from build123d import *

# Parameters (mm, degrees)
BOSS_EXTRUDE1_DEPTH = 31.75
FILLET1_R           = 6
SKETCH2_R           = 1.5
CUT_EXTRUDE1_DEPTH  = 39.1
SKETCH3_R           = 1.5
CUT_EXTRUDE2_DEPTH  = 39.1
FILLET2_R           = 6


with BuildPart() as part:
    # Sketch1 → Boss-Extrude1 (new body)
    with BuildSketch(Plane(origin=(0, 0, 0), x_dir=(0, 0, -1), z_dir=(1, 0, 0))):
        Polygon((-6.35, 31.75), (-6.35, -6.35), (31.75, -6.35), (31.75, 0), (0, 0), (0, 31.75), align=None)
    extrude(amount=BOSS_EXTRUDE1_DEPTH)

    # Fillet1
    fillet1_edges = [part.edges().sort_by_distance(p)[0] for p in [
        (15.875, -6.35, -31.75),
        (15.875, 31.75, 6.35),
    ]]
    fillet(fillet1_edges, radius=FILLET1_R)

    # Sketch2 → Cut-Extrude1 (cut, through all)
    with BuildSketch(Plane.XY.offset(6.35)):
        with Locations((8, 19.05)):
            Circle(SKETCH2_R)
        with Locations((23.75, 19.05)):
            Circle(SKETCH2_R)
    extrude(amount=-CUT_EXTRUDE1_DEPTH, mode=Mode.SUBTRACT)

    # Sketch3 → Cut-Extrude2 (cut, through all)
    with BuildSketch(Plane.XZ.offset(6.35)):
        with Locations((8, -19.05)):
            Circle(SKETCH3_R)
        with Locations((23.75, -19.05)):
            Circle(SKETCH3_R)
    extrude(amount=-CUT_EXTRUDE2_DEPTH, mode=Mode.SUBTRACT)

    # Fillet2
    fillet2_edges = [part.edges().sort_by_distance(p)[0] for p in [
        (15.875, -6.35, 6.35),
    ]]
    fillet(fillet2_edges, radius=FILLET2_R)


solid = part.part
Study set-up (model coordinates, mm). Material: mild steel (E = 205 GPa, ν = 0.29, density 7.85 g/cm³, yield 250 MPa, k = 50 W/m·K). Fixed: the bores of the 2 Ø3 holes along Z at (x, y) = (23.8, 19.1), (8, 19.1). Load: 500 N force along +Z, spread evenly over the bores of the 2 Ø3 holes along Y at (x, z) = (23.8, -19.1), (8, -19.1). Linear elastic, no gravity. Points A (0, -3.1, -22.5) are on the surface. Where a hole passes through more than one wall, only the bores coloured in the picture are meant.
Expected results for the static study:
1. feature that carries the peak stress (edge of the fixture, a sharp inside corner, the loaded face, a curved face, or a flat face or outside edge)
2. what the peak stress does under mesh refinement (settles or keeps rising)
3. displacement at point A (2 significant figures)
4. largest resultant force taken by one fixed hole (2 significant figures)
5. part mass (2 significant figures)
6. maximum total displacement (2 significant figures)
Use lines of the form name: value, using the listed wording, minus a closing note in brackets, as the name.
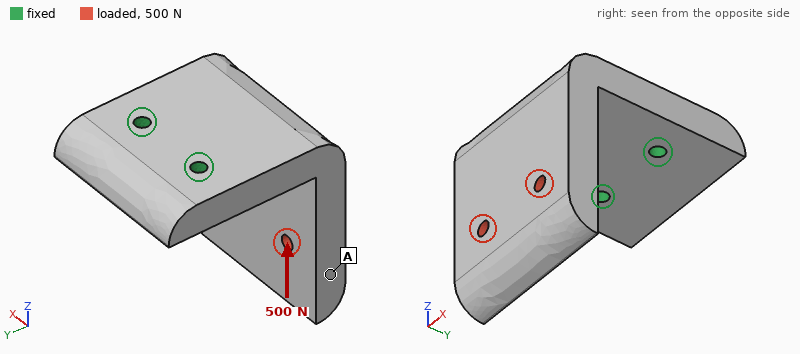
feature that carries the peak stress: edge of the fixture
what the peak stress does under mesh refinement: keeps rising
displacement at point A: 29 µm
largest resultant force taken by one fixed hole: 250 N
part mass: 100 g
maximum total displacement: 37 µm
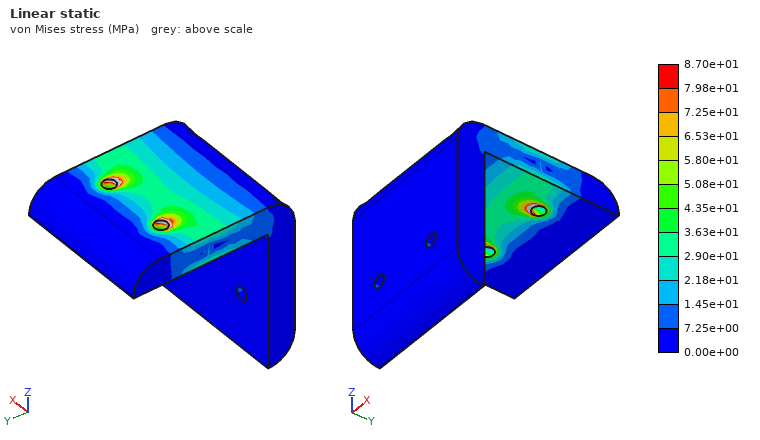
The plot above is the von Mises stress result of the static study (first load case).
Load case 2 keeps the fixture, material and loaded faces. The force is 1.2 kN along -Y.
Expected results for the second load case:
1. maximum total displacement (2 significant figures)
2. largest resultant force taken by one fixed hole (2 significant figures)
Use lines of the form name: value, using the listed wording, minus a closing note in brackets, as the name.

maximum total displacement: 0.20 mm
largest resultant force taken by one fixed hole: 610 N
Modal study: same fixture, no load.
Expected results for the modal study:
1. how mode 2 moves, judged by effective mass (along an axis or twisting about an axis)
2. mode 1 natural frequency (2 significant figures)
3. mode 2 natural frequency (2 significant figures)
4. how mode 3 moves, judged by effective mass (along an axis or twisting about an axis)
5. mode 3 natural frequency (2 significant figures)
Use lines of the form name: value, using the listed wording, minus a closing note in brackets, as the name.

how mode 2 moves, judged by effective mass: along X
mode 1 natural frequency: 2200 Hz
mode 2 natural frequency: 3600 Hz
how mode 3 moves, judged by effective mass: along Z
mode 3 natural frequency: 6200 Hz
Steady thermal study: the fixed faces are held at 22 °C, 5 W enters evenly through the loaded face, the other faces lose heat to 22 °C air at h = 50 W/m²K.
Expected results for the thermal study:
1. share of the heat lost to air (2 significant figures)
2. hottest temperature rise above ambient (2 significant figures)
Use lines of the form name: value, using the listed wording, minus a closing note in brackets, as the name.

share of the heat lost to air: 39 %
hottest temperature rise above ambient: 16 K
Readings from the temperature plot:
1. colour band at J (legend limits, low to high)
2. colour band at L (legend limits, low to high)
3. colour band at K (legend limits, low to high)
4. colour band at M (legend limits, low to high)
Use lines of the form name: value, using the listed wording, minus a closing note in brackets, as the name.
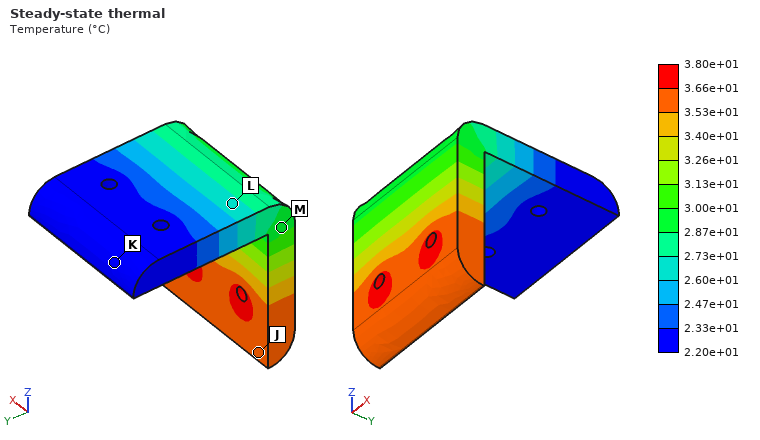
colour band at J: 3.53e+01 to 3.66e+01 °C
colour band at L: 2.60e+01 to 2.73e+01 °C
colour band at K: 2.20e+01 to 2.33e+01 °C
colour band at M: 2.87e+01 to 3.00e+01 °C
